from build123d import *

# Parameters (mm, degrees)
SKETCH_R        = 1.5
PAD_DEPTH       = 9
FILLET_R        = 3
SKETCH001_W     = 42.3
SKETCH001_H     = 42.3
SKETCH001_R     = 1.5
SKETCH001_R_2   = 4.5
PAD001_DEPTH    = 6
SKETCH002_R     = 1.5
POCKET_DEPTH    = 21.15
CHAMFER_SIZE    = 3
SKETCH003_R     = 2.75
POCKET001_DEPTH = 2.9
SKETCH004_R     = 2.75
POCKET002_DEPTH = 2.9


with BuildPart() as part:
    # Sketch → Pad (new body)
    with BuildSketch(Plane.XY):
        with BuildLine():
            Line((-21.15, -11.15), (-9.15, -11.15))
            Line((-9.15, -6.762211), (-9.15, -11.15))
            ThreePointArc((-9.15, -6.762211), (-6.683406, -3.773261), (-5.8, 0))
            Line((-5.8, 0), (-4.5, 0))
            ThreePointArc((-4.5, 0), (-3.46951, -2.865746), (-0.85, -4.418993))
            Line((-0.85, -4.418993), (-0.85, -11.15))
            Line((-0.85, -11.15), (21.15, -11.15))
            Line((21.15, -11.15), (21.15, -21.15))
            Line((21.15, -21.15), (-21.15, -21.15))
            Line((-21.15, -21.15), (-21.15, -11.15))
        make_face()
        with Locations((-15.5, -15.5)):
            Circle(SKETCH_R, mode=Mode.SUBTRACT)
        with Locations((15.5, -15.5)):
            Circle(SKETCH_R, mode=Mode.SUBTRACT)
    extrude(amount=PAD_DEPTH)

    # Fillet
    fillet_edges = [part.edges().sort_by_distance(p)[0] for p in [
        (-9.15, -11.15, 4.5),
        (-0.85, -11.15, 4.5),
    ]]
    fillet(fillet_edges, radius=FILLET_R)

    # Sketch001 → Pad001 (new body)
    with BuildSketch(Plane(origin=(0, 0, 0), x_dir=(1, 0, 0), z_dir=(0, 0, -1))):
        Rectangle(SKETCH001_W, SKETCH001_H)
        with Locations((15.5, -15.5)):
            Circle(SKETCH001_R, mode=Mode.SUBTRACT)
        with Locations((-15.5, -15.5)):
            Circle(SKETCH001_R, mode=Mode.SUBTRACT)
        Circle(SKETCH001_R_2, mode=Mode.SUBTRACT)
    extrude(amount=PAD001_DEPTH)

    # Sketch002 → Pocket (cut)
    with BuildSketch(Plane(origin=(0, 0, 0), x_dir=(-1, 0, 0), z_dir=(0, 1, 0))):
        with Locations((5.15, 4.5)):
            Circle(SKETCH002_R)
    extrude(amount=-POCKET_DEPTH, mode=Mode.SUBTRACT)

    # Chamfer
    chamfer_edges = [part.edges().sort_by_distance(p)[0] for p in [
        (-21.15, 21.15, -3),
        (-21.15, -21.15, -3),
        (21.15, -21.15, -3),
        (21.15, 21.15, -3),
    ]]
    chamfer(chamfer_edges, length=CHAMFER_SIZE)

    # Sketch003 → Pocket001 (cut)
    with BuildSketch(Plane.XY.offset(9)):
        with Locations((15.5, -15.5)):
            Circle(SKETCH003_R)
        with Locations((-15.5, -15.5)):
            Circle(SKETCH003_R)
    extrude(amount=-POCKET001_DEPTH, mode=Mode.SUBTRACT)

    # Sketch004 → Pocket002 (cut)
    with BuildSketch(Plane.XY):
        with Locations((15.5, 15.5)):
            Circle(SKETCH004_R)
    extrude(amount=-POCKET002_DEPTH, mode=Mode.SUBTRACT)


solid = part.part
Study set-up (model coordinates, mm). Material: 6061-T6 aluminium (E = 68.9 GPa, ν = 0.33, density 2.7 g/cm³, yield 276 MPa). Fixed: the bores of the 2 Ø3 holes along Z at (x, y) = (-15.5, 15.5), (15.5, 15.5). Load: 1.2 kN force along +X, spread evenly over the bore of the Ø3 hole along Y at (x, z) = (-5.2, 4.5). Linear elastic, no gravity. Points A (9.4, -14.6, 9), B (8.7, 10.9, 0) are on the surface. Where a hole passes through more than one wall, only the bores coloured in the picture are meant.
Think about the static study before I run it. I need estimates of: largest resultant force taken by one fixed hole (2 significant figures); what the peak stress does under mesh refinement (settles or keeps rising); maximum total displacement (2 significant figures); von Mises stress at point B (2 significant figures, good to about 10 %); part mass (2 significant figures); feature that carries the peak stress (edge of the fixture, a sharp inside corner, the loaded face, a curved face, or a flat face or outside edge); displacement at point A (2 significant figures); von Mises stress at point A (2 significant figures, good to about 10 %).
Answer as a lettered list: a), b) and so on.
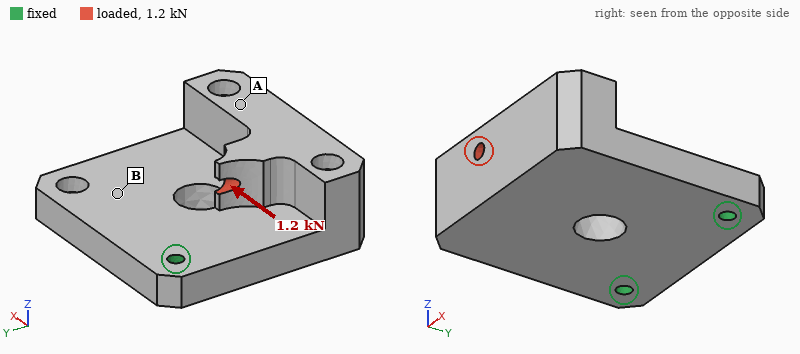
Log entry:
a) 1.3 kN
b) keeps rising
c) 52 µm
d) 21 MPa
e) 38 g
f) edge of the fixture
g) 37 µm
h) 8.4 MPa
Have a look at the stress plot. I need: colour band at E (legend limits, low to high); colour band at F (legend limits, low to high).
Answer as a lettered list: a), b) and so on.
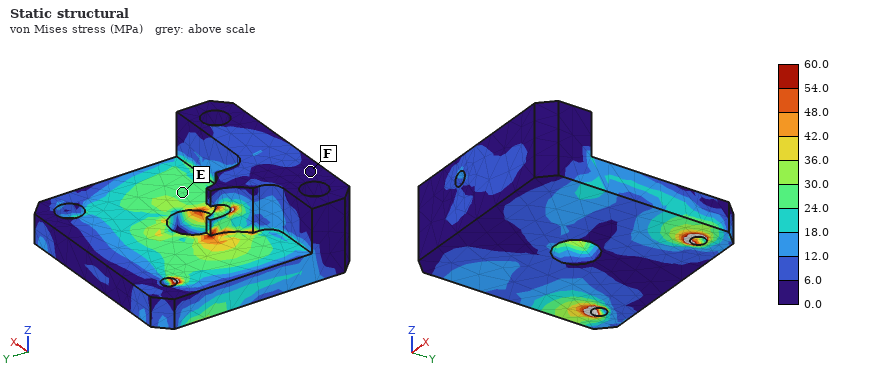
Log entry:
a) 24.0 to 30.0 MPa
b) 0.0 to 6.0 MPa
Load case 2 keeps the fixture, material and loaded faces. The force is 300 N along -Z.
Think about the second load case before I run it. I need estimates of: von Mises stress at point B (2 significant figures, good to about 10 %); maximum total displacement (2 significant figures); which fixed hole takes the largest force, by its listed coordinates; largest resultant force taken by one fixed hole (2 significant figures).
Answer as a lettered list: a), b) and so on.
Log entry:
a) 18 MPa
b) 0.11 mm
c) (-15.5, 15.5)
d) 220 N
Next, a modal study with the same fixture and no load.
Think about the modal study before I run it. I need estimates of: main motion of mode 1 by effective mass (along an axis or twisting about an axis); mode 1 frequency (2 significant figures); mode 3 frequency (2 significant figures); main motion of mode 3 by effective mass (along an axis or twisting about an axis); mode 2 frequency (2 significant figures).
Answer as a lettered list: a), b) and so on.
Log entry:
a) along Z
b) 1800 Hz
c) 9400 Hz
d) along X
e) 5500 Hz
